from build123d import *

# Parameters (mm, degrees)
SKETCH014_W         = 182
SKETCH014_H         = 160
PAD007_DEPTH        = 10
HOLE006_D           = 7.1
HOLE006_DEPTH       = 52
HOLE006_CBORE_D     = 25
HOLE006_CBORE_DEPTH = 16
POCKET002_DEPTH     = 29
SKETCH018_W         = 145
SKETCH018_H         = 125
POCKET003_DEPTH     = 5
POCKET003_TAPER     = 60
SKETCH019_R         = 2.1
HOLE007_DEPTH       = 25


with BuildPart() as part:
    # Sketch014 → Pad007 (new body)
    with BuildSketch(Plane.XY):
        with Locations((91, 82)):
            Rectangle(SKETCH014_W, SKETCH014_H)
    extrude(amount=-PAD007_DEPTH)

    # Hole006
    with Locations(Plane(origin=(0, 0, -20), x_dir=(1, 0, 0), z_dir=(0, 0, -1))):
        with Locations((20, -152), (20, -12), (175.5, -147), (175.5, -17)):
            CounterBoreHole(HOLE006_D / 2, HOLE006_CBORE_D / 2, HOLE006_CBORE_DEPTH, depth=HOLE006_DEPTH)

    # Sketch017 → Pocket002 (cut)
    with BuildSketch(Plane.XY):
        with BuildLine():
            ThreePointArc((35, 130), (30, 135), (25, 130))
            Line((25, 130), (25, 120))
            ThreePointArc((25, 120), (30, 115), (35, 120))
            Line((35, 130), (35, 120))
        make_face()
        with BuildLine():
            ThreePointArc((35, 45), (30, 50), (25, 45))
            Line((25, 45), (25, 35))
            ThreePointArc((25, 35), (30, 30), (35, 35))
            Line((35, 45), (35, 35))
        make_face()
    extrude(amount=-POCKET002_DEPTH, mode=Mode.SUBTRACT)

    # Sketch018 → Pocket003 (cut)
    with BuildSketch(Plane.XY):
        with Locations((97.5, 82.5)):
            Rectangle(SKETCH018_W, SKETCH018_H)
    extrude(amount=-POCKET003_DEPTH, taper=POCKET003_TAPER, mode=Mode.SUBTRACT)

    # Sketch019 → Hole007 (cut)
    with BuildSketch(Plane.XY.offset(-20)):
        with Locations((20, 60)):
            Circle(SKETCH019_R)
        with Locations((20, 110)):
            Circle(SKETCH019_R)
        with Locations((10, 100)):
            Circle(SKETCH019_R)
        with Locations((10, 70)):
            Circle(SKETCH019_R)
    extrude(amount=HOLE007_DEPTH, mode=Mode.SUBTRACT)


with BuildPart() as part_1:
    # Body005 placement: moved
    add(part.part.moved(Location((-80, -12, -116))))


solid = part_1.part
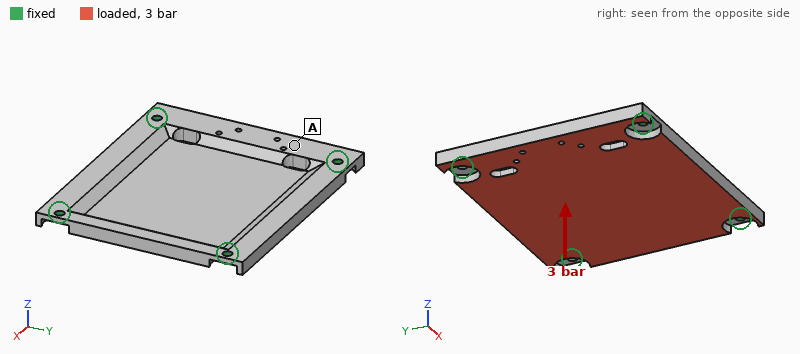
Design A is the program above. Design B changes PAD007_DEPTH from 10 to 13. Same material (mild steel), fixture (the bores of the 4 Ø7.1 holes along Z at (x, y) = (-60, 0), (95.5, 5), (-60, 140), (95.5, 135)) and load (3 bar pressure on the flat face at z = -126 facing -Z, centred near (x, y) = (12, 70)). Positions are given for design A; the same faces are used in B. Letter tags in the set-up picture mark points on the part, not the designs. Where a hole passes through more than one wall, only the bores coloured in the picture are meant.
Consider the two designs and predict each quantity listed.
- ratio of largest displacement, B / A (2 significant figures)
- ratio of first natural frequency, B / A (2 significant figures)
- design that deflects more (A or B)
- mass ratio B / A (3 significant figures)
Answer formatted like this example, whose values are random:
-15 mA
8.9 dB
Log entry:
0.43
1.2
A
1.41
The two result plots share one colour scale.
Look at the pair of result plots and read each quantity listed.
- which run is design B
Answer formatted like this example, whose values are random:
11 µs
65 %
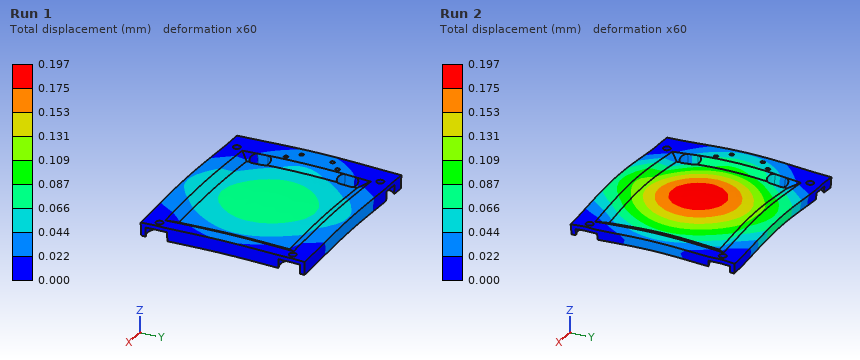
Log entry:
Run 1
